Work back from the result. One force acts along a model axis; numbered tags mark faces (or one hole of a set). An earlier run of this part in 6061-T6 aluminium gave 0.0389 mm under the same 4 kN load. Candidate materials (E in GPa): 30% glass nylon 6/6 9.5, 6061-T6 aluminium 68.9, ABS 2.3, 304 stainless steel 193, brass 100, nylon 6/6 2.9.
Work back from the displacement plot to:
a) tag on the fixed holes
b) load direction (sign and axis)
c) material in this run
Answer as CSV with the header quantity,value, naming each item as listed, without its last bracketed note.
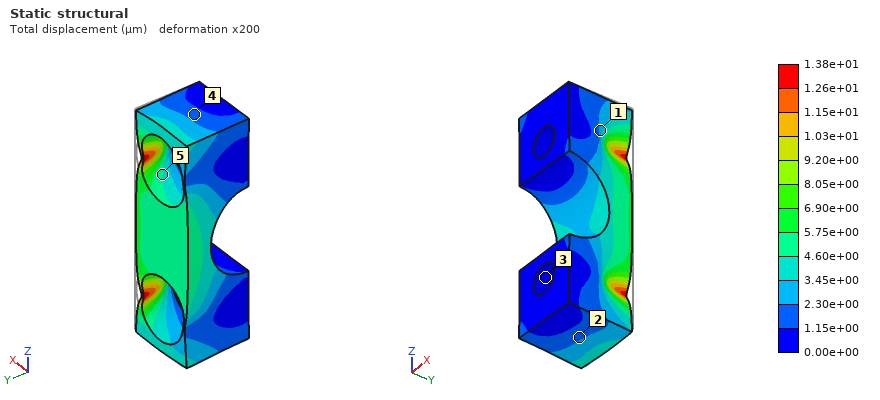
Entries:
quantity,value
tag on the fixed holes,3
load direction,-X
material in this run,304 stainless steel
